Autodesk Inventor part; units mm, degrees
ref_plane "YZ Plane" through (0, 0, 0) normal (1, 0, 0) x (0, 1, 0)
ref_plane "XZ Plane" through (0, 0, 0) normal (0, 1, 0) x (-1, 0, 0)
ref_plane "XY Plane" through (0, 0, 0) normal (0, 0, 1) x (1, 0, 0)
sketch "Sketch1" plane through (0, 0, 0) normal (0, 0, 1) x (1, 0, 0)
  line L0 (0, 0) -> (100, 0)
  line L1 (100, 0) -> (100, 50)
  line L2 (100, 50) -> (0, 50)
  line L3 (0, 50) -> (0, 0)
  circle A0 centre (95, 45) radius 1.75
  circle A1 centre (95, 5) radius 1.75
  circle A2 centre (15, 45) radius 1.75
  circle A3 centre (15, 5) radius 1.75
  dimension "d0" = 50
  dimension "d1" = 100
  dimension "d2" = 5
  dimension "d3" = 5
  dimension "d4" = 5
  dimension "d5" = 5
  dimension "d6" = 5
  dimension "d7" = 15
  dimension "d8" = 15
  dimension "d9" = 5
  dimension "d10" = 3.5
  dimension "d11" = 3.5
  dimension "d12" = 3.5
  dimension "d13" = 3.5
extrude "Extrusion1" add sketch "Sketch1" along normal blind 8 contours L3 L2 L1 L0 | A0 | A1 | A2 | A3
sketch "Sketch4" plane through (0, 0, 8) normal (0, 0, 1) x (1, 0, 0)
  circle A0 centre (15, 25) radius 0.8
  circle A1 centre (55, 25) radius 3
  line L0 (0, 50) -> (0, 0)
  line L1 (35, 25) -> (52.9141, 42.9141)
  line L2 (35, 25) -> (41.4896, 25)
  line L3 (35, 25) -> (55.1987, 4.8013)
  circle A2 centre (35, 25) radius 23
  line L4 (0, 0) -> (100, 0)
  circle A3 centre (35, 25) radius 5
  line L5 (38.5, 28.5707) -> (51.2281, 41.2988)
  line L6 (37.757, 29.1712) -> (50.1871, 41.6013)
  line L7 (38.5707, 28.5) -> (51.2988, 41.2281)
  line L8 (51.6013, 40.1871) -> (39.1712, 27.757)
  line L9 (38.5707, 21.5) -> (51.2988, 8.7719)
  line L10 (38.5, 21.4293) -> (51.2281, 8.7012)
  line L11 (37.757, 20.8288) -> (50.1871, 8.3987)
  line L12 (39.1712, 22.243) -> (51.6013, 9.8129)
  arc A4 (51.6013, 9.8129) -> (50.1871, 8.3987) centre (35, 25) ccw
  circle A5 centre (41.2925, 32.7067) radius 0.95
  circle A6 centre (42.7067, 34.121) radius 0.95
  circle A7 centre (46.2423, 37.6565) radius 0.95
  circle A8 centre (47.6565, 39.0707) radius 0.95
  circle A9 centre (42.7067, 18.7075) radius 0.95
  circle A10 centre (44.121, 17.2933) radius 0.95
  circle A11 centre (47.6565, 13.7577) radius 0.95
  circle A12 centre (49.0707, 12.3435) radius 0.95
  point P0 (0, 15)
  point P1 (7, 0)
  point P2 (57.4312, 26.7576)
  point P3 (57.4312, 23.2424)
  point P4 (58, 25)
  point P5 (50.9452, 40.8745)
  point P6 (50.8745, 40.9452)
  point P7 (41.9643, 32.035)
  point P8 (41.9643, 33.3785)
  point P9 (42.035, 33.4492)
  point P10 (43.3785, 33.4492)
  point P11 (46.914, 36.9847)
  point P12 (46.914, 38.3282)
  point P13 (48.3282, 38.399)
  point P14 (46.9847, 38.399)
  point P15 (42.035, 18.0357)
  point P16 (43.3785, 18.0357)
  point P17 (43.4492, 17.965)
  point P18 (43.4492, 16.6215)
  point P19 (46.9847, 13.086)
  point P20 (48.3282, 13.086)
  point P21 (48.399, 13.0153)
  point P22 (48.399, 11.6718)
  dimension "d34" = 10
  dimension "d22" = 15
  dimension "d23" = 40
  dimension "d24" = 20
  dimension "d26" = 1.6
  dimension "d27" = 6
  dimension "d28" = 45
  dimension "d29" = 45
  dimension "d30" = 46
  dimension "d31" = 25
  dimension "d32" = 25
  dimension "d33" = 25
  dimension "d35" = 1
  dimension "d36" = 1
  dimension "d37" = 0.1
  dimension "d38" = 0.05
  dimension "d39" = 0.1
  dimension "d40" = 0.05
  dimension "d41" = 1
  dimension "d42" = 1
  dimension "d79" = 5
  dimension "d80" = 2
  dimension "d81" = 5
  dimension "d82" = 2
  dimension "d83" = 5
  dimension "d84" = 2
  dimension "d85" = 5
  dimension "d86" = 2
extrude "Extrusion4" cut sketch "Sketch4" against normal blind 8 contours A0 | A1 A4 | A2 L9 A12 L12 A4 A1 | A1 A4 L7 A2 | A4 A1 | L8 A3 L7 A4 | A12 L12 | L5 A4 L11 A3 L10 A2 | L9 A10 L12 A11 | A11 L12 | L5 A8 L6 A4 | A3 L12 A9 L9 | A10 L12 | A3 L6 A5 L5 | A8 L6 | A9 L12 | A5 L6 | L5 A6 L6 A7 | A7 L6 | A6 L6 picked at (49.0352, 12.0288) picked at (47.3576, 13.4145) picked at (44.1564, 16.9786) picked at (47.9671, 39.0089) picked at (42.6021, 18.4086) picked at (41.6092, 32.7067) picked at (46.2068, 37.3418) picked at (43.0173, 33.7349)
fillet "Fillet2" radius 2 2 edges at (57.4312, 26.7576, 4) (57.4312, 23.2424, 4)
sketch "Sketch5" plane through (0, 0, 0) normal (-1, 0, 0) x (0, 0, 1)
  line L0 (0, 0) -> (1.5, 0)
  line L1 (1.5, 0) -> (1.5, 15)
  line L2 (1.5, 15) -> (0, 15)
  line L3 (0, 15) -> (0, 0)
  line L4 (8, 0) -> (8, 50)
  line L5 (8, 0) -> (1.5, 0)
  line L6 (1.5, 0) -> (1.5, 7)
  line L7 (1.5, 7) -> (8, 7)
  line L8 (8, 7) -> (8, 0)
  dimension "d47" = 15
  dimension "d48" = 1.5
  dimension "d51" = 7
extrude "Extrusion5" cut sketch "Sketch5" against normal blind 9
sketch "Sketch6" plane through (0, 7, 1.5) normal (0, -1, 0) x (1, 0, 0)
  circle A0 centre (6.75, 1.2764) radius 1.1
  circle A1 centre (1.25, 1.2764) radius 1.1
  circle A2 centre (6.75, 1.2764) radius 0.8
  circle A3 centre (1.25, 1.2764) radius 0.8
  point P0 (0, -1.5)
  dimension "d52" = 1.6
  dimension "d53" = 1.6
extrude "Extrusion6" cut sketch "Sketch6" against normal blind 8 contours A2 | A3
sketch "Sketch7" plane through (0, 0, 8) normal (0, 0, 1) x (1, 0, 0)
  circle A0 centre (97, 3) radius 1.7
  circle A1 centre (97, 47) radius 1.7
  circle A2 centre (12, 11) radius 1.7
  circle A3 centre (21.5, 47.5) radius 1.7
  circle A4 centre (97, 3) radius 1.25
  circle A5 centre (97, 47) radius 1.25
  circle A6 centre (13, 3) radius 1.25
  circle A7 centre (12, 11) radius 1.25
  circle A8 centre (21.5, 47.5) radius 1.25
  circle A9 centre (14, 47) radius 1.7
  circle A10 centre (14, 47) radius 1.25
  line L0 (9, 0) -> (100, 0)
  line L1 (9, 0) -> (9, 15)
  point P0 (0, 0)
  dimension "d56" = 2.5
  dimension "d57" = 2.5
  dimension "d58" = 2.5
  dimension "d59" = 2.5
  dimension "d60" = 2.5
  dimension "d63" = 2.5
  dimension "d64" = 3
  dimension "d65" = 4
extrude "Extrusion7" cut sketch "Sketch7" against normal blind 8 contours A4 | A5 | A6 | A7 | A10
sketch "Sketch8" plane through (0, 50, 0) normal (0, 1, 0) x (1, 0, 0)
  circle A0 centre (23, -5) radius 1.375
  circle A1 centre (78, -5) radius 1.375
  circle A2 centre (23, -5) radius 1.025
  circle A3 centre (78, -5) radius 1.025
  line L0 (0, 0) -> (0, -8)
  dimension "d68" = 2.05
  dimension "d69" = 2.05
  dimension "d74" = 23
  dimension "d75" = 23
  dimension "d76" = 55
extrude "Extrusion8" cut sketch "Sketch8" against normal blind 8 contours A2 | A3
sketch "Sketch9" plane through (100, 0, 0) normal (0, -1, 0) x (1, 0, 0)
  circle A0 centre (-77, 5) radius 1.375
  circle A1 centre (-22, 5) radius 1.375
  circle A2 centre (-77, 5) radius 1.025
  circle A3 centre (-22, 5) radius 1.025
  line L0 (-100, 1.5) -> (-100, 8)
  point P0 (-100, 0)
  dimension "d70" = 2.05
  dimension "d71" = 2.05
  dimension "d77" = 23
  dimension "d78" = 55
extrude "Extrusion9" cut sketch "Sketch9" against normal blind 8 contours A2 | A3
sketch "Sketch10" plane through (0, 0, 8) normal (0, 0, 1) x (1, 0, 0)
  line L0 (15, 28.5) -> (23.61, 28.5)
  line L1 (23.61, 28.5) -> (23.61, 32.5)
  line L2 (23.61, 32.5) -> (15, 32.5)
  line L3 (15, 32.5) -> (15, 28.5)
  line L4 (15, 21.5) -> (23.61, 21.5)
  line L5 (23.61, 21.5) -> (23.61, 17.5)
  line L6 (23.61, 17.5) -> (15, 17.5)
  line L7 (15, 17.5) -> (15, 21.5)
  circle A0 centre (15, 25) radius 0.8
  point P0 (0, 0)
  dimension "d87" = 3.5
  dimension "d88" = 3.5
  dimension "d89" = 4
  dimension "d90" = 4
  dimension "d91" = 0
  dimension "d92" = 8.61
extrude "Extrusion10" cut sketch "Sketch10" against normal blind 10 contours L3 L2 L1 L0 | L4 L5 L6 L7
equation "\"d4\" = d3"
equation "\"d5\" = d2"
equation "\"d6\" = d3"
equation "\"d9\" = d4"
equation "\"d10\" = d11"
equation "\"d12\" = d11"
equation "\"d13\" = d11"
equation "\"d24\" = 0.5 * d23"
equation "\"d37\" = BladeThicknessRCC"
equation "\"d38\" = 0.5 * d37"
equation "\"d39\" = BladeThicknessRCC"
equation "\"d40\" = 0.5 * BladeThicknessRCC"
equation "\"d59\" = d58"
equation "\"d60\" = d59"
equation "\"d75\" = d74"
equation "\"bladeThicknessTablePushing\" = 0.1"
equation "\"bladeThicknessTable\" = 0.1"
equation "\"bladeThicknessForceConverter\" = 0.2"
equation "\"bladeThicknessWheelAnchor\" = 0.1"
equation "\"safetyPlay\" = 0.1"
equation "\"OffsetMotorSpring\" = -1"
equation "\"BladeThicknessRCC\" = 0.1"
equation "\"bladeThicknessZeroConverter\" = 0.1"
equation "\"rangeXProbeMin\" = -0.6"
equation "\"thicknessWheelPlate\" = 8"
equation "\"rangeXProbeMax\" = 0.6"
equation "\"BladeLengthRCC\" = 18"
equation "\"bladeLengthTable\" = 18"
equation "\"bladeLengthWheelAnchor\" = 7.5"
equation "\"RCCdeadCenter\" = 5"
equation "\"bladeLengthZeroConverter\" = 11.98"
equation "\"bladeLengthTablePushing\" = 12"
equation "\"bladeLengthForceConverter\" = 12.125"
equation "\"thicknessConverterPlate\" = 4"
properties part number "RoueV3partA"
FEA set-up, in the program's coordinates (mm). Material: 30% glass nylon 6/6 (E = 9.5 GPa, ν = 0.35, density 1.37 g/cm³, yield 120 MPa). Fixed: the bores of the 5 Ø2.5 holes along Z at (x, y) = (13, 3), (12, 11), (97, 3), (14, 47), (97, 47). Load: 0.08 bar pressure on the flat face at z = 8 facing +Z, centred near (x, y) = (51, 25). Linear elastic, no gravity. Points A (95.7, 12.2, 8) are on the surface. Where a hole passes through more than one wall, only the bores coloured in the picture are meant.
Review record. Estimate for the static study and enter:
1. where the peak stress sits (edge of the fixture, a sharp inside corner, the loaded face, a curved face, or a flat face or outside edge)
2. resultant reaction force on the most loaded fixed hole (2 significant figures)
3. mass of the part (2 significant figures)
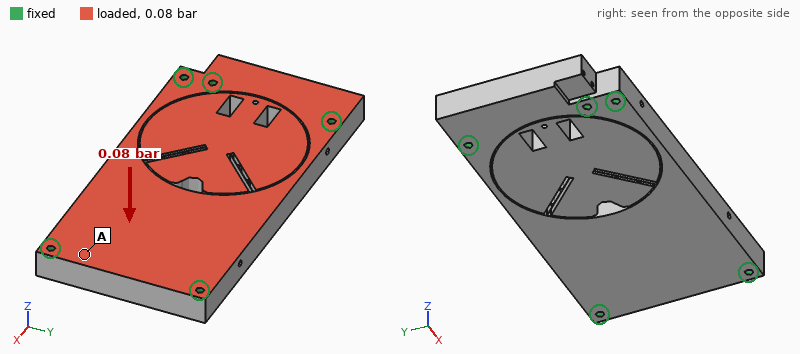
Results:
a flat face or outside edge
10 N
51 g
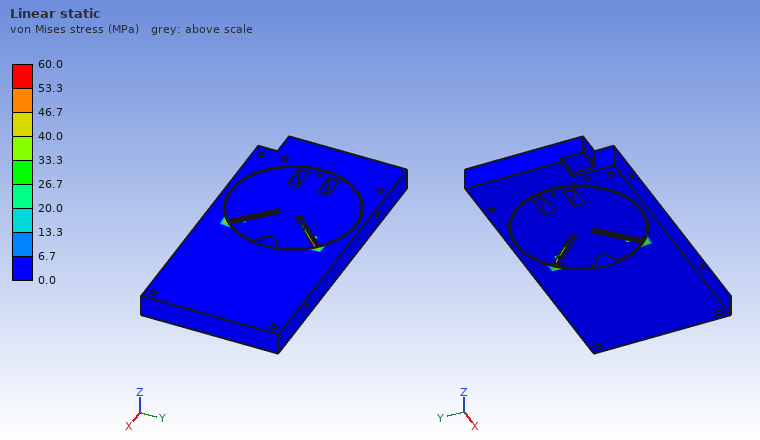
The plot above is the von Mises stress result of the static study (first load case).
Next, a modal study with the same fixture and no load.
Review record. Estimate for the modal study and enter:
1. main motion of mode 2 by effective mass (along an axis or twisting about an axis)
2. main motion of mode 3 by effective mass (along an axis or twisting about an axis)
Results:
along Z
along Y
